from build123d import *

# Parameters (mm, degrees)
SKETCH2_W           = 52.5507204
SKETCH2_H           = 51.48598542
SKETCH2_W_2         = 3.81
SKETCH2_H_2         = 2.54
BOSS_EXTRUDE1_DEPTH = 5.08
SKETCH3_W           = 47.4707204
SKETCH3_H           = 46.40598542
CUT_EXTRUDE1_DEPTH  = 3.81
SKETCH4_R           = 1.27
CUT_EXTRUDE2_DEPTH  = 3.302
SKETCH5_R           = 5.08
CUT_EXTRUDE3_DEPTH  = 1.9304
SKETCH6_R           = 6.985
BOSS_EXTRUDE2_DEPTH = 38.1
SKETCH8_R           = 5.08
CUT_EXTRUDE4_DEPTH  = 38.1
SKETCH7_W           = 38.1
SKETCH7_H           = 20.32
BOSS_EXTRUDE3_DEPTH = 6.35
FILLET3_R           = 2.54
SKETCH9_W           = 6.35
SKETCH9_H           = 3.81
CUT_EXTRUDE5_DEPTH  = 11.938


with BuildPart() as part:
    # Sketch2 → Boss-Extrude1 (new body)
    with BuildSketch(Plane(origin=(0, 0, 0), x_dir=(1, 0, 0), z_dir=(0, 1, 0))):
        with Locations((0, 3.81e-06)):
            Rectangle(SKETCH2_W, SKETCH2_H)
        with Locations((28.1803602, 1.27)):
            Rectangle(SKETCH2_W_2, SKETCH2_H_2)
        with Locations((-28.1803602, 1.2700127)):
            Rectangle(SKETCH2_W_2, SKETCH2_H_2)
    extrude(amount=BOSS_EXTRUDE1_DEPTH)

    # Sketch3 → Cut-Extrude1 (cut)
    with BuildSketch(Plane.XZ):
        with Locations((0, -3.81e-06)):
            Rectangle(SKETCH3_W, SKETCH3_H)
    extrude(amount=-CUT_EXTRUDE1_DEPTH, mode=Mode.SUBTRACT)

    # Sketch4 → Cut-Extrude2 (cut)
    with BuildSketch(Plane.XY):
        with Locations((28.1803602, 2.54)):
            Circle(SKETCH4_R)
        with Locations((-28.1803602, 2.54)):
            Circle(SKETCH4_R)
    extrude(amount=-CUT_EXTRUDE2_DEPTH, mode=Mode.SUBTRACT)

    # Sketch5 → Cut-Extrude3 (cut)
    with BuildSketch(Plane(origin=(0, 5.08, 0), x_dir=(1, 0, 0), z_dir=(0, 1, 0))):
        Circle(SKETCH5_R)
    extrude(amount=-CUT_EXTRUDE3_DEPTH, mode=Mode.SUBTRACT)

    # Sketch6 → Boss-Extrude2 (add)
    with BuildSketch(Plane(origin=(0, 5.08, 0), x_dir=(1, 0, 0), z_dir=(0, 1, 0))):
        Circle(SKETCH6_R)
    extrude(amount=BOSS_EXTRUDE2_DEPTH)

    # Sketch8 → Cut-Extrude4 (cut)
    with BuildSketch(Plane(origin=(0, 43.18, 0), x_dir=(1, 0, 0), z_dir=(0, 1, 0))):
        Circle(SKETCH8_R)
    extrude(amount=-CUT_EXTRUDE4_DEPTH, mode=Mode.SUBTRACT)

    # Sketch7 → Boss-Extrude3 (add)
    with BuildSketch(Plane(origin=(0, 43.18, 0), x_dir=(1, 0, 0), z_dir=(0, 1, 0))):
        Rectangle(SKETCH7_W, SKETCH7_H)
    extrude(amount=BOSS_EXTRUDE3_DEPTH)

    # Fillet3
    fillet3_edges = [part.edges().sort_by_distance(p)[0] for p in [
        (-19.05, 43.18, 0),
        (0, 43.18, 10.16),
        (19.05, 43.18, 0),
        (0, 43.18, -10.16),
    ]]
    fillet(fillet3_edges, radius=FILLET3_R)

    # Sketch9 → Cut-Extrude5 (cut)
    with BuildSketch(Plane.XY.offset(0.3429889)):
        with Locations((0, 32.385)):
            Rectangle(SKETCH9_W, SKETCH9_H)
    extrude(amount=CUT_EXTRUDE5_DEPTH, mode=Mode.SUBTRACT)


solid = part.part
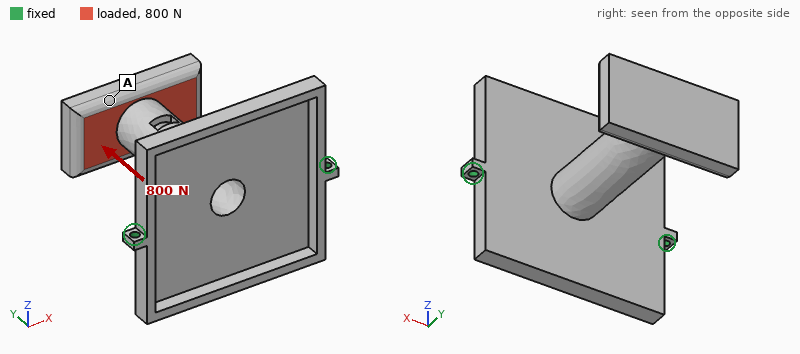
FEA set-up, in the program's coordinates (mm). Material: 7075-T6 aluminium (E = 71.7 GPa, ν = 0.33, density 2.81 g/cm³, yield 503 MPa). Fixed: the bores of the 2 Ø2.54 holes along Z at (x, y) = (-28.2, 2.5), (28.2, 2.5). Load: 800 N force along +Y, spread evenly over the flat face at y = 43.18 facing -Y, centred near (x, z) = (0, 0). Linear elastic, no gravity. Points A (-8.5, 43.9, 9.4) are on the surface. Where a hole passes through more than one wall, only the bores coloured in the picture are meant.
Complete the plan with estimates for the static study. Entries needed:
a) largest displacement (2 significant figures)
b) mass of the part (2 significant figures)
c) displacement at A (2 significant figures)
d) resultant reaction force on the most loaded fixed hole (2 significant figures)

0.56 mm
36 g
0.55 mm
690 N
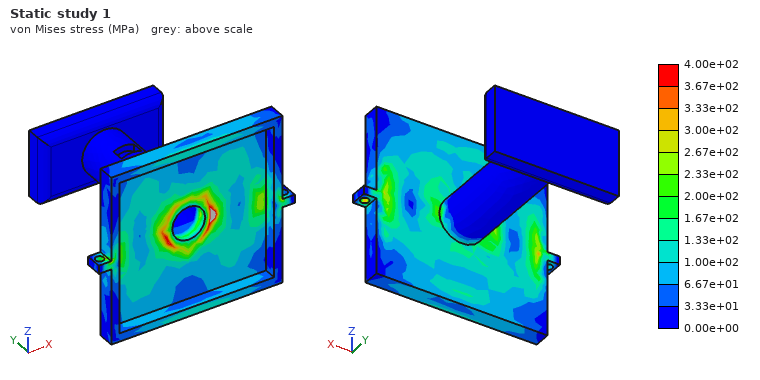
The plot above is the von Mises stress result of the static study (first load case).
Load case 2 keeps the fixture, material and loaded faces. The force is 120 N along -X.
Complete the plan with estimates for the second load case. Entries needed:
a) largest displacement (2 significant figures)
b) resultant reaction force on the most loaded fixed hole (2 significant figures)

0.79 mm
130 N
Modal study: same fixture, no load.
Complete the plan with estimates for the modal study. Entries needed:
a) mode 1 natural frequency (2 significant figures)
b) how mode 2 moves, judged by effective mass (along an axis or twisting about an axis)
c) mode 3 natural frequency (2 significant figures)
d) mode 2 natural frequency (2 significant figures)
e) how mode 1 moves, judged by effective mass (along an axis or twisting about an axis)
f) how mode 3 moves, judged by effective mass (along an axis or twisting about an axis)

380 Hz
along X
1300 Hz
500 Hz
along Z
along Y
